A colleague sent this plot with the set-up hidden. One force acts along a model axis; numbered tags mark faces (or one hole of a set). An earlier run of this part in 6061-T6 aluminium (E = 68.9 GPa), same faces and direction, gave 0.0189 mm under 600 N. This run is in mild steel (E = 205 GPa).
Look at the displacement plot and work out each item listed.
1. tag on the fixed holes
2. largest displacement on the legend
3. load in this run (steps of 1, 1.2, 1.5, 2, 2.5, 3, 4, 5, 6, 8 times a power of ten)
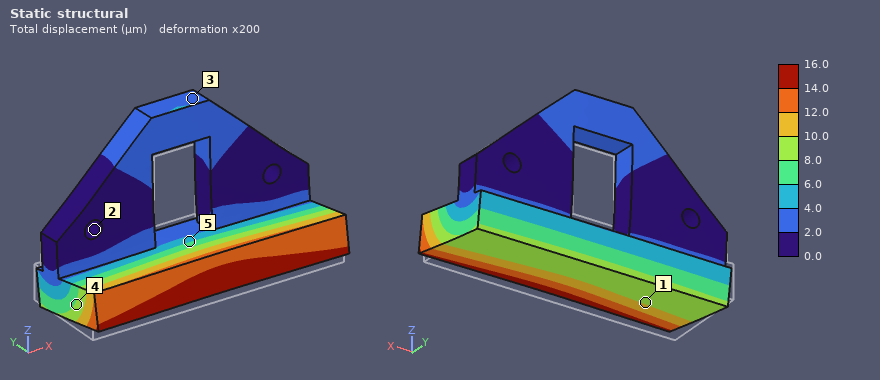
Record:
2
16.0 µm
1.5 kN
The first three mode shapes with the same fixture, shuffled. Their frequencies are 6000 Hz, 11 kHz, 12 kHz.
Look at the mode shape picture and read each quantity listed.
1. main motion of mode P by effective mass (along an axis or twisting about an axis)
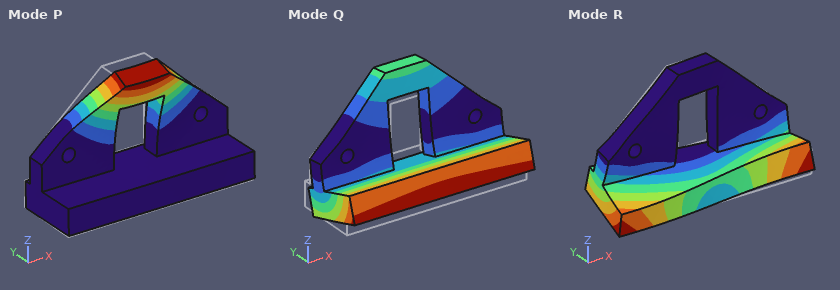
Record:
along Y
